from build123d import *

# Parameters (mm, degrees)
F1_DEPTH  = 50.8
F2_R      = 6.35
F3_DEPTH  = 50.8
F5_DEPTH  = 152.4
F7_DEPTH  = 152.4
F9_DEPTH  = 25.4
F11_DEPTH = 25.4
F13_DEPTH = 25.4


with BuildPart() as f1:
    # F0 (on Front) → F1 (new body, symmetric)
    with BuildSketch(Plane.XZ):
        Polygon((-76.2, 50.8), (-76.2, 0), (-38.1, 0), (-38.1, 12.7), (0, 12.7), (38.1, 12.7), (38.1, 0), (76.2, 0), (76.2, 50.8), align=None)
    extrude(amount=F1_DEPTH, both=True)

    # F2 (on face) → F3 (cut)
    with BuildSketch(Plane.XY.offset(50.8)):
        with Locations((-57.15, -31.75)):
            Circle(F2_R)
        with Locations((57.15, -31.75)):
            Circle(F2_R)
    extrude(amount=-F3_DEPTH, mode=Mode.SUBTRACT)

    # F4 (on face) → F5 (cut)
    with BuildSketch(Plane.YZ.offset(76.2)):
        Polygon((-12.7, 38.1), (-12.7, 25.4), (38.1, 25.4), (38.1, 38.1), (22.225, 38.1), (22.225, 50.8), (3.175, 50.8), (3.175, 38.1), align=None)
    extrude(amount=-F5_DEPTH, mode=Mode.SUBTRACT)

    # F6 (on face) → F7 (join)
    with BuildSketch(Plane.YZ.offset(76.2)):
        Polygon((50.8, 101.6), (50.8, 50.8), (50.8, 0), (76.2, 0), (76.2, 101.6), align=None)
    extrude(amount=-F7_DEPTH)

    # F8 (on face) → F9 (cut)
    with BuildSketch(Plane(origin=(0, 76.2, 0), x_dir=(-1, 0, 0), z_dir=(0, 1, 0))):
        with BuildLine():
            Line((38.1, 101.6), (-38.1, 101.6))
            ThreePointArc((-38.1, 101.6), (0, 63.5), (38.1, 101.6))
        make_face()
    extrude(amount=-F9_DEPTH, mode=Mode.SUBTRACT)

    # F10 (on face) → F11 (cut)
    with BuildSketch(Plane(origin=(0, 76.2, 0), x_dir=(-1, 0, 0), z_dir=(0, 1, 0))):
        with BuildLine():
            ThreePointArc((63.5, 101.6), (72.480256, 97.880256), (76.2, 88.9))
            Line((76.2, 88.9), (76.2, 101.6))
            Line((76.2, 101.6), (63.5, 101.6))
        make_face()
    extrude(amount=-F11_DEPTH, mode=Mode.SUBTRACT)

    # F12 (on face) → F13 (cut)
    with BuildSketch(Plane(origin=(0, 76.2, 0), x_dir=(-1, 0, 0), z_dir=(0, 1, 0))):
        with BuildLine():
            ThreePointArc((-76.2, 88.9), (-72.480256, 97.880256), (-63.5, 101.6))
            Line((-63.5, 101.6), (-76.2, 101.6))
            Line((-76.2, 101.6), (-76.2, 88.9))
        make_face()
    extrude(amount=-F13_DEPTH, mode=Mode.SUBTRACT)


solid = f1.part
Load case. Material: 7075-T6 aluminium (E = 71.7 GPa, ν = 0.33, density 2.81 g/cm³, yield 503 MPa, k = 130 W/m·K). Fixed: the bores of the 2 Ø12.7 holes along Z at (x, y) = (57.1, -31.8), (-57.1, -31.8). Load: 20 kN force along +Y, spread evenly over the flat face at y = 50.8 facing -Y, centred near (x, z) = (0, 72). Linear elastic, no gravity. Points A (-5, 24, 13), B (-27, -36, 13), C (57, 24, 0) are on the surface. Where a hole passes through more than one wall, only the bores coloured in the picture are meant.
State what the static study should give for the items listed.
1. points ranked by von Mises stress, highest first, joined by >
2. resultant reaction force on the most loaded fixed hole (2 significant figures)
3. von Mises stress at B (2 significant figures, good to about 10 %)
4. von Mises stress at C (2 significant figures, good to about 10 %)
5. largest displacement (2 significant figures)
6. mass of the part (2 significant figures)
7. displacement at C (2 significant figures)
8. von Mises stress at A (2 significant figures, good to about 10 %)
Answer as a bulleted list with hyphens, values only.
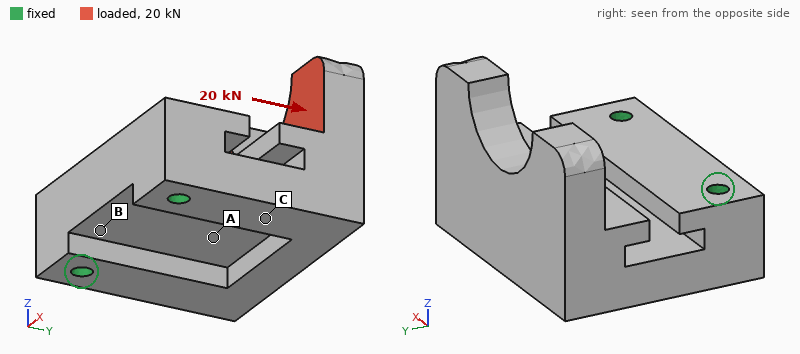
- C > A > B
- 12 kN
- 16 MPa
- 110 MPa
- 0.99 mm
- 2.5 kg
- 0.15 mm
- 51 MPa
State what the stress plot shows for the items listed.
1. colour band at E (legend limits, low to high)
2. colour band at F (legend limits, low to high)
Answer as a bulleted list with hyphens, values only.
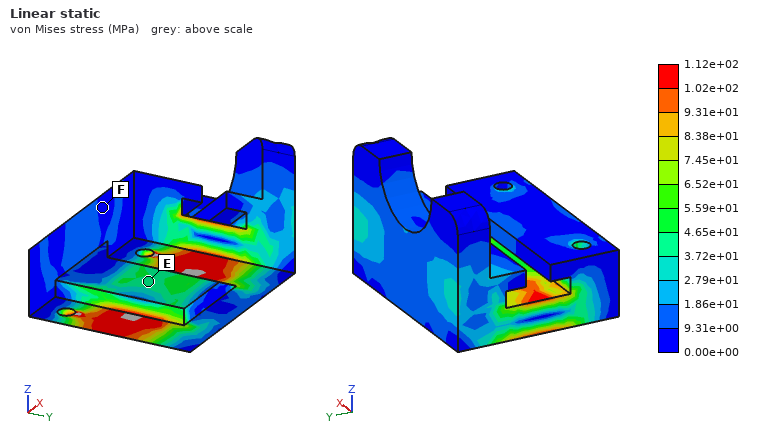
- 3.72e+01 to 4.65e+01 MPa
- 0.00e+00 to 9.31e+00 MPa
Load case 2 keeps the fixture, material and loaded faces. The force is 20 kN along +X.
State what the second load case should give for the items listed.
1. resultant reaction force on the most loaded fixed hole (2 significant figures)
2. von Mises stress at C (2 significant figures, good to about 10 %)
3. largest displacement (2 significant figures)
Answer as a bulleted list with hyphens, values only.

- 18 kN
- 25 MPa
- 0.28 mm
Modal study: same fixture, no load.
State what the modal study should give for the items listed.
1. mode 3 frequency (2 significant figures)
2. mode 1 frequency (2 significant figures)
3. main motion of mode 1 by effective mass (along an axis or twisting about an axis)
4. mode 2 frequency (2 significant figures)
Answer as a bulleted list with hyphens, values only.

- 2900 Hz
- 820 Hz
- along Z
- 1700 Hz
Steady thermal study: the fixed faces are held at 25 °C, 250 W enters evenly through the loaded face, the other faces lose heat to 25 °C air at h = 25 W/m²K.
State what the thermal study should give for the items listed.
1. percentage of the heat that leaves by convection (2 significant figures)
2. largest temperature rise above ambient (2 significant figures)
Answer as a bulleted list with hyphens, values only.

- 25 %
- 67 K
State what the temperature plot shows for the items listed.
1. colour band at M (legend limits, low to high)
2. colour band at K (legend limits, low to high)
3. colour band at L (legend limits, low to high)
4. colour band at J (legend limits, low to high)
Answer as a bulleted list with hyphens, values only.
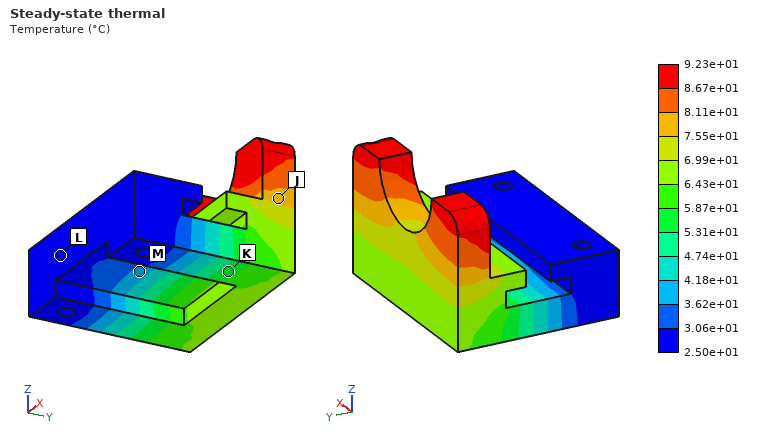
- 3.62e+01 to 4.18e+01 °C
- 5.31e+01 to 5.87e+01 °C
- 2.50e+01 to 3.06e+01 °C
- 7.55e+01 to 8.11e+01 °C
